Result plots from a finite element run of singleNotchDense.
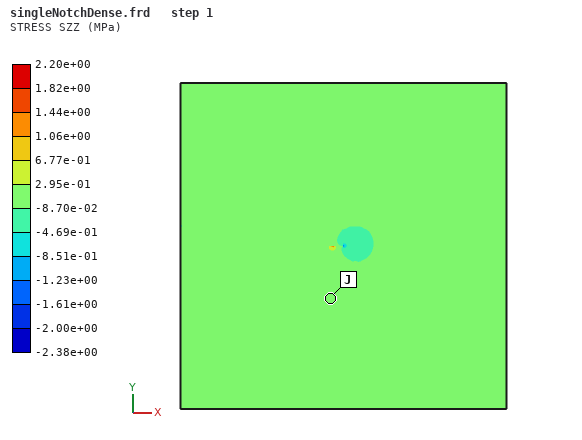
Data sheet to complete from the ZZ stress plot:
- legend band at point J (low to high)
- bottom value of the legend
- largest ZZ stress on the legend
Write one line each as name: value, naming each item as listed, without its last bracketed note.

legend band at point J: -8.70e-02 to 2.95e-01 MPa
bottom value of the legend: -2.38e+00 MPa
largest ZZ stress on the legend: 2.20e+00 MPa
